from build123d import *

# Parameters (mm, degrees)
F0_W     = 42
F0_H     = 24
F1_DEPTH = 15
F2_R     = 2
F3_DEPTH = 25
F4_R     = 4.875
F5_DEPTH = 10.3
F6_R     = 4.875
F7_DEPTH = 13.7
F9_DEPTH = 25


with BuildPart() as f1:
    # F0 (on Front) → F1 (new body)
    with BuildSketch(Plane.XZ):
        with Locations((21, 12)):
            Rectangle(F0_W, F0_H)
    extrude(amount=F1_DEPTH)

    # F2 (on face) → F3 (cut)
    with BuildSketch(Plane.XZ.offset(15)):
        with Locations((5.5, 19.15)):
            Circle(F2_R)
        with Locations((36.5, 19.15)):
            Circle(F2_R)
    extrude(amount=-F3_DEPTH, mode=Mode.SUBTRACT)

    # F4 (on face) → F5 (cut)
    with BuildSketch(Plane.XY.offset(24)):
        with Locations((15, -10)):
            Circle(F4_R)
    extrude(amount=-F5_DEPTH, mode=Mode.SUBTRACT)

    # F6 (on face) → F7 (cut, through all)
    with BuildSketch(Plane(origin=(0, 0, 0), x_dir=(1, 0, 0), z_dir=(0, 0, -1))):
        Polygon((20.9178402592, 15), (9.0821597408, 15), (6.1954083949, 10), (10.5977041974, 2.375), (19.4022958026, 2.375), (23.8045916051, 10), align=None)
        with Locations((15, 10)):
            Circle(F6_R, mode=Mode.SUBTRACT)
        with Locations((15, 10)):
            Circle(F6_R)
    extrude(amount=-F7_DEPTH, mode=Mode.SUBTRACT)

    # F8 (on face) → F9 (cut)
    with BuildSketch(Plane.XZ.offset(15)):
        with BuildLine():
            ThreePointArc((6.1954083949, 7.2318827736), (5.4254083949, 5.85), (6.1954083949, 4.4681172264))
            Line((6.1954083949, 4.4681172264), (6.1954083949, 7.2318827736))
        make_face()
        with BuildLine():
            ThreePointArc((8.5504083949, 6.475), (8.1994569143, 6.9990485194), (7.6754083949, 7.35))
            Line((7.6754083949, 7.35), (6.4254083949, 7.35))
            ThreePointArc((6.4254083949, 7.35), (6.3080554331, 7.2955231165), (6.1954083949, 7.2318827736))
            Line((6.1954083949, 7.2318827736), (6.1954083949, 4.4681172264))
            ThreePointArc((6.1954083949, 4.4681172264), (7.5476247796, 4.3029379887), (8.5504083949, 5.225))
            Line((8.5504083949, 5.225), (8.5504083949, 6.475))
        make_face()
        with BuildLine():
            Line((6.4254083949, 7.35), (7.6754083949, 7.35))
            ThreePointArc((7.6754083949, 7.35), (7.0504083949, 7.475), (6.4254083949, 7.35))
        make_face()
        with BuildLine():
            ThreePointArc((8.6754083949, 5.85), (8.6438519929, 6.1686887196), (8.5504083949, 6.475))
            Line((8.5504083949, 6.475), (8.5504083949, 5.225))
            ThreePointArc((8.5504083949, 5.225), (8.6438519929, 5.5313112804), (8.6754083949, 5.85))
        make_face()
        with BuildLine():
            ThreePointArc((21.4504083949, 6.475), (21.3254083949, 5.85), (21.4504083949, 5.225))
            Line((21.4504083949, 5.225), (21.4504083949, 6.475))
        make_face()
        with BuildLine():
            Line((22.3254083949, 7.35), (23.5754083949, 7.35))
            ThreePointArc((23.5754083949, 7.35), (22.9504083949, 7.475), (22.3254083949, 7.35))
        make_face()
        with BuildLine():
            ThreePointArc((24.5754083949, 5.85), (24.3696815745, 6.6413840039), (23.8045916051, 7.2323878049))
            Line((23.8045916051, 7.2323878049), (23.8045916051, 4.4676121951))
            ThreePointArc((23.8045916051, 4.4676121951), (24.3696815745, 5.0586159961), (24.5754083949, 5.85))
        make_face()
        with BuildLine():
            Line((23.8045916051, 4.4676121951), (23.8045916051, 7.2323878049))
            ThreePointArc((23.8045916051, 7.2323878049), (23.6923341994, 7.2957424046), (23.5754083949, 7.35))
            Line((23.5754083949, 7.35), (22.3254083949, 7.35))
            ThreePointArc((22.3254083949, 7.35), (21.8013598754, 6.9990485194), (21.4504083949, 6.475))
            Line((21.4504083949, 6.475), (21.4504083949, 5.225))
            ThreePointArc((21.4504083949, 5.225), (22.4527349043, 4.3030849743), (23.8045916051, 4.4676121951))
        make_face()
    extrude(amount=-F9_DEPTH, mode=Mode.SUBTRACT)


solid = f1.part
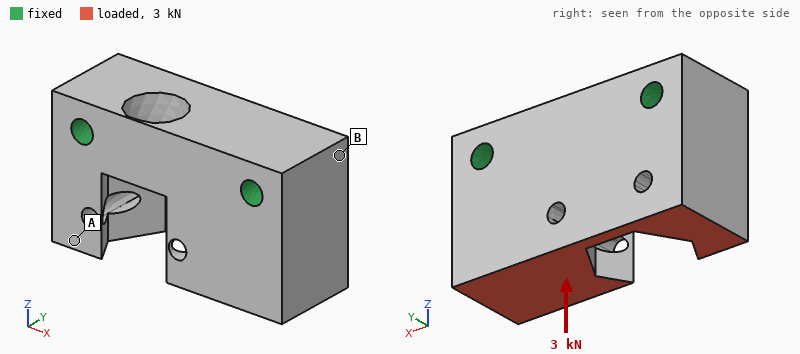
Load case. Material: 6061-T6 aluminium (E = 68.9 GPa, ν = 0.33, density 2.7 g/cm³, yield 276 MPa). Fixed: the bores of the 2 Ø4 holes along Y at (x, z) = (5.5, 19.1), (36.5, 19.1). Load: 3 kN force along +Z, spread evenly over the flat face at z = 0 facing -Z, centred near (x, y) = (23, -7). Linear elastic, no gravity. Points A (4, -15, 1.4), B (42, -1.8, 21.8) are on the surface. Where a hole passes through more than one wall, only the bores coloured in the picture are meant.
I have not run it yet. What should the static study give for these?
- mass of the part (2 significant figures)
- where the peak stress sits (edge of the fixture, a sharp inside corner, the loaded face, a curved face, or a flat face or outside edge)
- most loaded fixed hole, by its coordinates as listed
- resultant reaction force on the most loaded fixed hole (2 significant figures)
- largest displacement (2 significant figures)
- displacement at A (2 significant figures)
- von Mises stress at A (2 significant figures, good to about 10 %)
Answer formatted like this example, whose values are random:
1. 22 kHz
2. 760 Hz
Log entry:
1. 31 g
2. a curved face
3. (36.5, 19.1)
4. 1.8 kN
5. 6.2 µm
6. 2.0 µm
7. 8.2 MPa
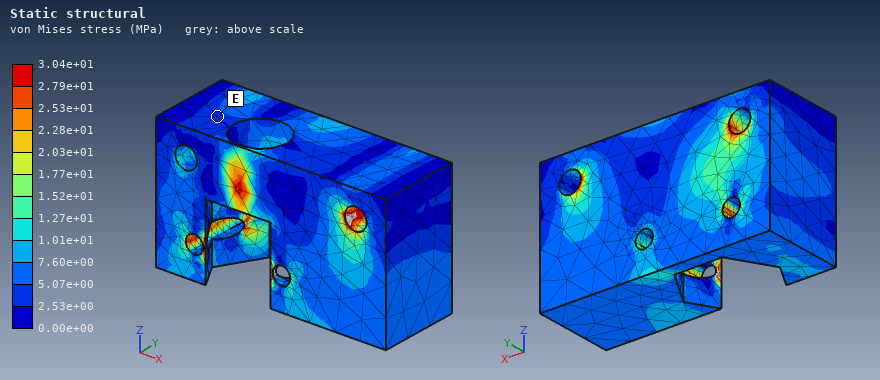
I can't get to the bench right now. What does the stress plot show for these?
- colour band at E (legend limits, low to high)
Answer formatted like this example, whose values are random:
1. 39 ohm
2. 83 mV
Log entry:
1. 2.53e+00 to 5.07e+00 MPa
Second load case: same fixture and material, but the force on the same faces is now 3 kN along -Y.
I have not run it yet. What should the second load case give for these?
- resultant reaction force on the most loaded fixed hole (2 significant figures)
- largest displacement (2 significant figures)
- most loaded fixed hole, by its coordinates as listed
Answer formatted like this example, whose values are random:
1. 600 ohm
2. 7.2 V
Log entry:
1. 2.0 kN
2. 35 µm
3. (36.5, 19.1)
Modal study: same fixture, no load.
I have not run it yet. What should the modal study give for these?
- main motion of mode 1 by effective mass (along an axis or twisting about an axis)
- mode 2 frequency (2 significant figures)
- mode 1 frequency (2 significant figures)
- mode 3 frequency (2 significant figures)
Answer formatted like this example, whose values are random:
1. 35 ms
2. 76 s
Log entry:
1. along Y
2. 21 kHz
3. 19 kHz
4. 25 kHz
